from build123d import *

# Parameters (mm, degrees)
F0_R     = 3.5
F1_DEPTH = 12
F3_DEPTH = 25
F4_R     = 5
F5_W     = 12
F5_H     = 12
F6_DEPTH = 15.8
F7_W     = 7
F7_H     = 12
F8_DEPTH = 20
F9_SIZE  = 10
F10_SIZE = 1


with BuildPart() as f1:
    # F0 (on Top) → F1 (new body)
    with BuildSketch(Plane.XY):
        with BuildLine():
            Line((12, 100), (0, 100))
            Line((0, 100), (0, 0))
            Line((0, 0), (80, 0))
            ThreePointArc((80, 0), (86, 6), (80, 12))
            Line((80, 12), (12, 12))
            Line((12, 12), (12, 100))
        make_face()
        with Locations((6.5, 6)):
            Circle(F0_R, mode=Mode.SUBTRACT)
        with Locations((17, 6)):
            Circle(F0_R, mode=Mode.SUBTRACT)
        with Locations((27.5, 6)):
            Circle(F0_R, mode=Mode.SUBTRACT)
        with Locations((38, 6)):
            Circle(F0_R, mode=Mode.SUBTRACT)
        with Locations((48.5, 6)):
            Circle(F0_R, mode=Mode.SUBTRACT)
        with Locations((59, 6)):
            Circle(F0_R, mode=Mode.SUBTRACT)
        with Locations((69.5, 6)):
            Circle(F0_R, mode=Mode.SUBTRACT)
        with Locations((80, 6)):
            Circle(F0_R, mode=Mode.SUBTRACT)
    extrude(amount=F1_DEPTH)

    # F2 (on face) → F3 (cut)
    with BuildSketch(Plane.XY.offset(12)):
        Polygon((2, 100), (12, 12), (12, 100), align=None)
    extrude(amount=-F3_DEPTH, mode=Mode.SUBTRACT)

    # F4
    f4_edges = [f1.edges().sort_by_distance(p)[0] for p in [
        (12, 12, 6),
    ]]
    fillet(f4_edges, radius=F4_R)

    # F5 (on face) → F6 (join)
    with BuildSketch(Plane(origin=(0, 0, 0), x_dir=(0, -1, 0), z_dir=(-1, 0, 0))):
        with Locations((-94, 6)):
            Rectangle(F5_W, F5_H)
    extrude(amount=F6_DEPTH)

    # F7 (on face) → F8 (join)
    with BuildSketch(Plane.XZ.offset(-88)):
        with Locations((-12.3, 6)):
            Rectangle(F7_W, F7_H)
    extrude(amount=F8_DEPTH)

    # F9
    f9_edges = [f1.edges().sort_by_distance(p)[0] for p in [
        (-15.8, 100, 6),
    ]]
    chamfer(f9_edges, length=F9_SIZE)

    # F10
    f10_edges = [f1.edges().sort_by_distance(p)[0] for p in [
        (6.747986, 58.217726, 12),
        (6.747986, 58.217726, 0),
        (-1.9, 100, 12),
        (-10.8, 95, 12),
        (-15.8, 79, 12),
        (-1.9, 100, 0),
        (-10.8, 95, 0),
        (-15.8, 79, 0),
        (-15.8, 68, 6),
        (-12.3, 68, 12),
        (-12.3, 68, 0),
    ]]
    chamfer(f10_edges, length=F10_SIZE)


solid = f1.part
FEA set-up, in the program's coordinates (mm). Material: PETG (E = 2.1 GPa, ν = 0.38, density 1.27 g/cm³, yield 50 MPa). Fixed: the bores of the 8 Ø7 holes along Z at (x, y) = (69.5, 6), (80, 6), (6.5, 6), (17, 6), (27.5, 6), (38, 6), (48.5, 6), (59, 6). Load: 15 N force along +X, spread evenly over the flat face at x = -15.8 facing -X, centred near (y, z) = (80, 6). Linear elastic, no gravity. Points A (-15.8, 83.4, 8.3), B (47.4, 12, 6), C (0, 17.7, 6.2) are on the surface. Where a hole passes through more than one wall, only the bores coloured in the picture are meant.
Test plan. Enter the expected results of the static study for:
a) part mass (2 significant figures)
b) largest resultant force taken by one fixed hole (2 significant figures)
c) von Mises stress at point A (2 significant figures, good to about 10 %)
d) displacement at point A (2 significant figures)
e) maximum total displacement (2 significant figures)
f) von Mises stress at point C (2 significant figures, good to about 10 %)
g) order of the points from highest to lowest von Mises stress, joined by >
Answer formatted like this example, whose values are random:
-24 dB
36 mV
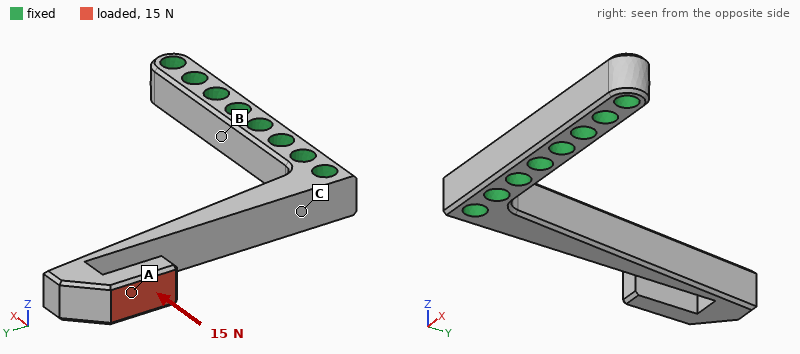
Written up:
24 g
82 N
0.82 MPa
1.2 mm
1.4 mm
3.6 MPa
C > A > B
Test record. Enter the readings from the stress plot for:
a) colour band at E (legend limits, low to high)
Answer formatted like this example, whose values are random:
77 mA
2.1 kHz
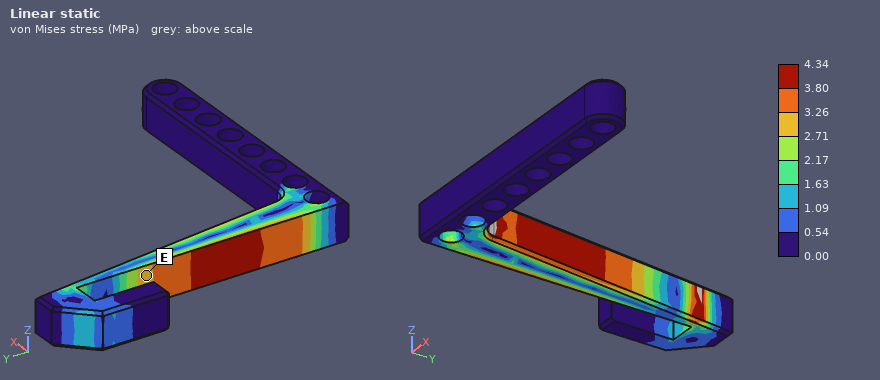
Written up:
2.71 to 3.26 MPa
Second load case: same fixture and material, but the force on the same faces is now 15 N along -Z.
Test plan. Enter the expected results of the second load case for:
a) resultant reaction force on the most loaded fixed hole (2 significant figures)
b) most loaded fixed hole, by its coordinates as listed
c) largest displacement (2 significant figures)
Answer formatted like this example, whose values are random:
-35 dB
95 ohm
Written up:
23 N
(6.5, 6)
1.6 mm
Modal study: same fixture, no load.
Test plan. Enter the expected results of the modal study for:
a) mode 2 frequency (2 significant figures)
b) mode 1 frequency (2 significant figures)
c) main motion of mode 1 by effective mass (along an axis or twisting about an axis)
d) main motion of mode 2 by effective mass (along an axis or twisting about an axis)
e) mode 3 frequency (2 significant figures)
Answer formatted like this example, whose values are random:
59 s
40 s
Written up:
250 Hz
200 Hz
along X
along Z
470 Hz
